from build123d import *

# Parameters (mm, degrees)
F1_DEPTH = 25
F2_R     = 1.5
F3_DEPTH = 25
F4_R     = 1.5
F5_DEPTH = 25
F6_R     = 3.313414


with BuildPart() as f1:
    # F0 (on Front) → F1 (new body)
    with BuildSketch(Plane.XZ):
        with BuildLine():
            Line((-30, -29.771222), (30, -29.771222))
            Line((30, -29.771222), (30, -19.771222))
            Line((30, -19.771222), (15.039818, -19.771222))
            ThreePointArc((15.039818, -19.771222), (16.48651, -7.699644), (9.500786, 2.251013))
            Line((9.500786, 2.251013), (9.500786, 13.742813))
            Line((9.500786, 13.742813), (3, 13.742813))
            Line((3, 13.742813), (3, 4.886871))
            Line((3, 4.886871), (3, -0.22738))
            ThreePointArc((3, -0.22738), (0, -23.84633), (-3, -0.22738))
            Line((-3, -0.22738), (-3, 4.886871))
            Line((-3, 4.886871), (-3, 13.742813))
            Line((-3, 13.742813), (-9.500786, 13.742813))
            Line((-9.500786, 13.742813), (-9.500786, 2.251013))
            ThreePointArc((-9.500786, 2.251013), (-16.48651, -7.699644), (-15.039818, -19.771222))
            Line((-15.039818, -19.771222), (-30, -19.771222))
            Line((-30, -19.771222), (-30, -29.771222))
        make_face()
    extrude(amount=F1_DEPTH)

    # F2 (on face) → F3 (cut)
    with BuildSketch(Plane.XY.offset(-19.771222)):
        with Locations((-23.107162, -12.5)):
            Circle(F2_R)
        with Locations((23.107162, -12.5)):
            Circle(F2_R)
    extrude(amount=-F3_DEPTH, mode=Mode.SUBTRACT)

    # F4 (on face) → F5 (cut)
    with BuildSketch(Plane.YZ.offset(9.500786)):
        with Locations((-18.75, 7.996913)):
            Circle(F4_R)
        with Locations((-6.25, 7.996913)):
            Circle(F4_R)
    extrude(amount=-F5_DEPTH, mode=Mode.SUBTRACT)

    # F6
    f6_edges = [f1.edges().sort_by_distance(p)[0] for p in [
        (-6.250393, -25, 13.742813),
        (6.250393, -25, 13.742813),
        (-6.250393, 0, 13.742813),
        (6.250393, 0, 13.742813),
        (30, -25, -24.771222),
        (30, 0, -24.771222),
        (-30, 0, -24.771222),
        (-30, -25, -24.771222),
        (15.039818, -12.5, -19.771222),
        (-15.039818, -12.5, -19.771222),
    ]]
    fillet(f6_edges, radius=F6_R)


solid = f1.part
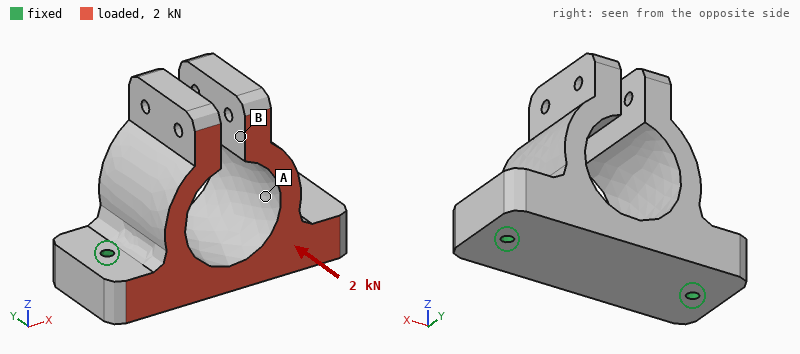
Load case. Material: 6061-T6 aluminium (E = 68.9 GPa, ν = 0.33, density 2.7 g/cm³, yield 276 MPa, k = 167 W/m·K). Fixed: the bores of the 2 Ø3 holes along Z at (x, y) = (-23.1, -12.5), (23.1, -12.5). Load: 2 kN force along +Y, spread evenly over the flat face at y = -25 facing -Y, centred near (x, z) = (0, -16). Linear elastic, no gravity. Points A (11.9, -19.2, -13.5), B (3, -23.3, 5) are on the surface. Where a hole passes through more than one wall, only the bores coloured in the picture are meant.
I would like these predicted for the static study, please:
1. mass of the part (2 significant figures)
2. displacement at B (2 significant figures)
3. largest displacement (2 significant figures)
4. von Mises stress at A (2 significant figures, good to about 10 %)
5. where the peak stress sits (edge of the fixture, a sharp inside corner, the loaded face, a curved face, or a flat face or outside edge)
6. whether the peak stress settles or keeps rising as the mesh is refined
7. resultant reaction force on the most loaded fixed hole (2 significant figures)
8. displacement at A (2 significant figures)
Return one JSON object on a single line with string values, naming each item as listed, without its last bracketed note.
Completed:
{"mass of the part": "64 g", "displacement at B": "35 µm", "largest displacement": "41 µm", "von Mises stress at A": "13 MPa", "where the peak stress sits": "edge of the fixture", "whether the peak stress settles or keeps rising as the mesh is refined": "keeps rising", "resultant reaction force on the most loaded fixed hole": "1.0 kN", "displacement at A": "13 µm"}
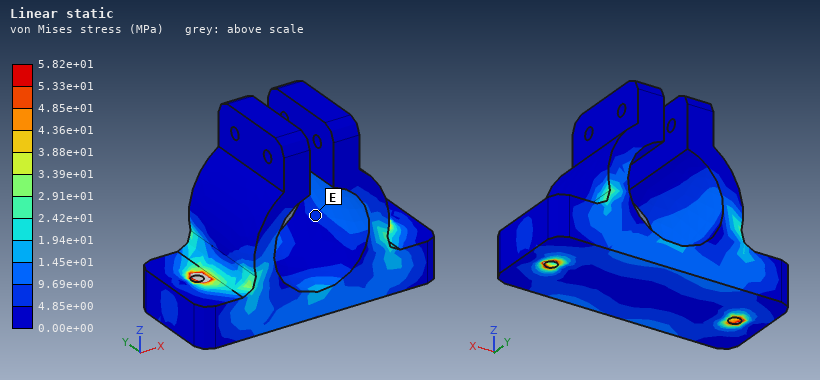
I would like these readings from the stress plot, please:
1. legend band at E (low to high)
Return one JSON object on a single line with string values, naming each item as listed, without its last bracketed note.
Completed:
{"legend band at E": "4.85e+00 to 9.69e+00 MPa"}
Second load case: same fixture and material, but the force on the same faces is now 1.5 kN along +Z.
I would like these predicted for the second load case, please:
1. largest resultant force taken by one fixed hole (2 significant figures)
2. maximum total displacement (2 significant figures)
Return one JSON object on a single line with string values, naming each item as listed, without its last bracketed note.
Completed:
{"largest resultant force taken by one fixed hole": "780 N", "maximum total displacement": "63 µm"}
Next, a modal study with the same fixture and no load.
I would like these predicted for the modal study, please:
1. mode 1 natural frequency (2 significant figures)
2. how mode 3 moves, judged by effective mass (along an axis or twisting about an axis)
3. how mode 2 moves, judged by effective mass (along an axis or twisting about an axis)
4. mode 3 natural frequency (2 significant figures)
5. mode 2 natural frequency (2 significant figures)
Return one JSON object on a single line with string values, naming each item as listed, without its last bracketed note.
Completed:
{"mode 1 natural frequency": "2900 Hz", "how mode 3 moves, judged by effective mass": "along Y", "how mode 2 moves, judged by effective mass": "along X", "mode 3 natural frequency": "5100 Hz", "mode 2 natural frequency": "3100 Hz"}
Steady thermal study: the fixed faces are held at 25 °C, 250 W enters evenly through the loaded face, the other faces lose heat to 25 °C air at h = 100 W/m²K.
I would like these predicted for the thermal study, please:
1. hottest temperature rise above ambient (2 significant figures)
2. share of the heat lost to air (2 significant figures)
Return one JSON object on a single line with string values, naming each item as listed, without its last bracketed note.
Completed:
{"hottest temperature rise above ambient": "74 K", "share of the heat lost to air": "13 %"}
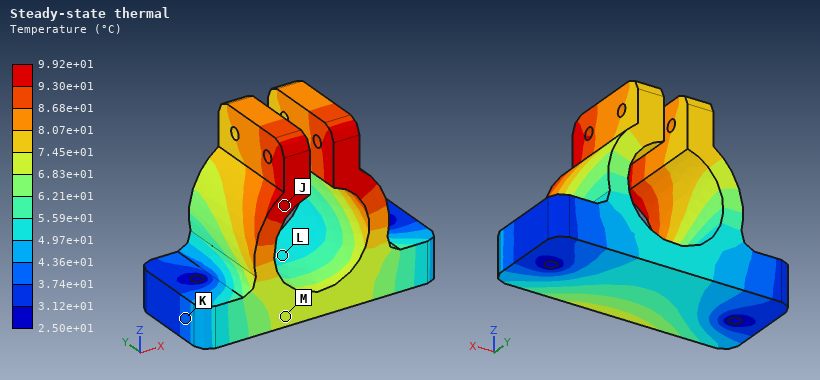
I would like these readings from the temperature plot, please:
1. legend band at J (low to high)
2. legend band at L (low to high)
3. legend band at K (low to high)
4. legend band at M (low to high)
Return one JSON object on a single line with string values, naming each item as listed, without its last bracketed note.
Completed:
{"legend band at J": "9.30e+01 to 9.92e+01 °C", "legend band at L": "4.97e+01 to 5.59e+01 °C", "legend band at K": "3.74e+01 to 4.36e+01 °C", "legend band at M": "6.83e+01 to 7.45e+01 °C"}
